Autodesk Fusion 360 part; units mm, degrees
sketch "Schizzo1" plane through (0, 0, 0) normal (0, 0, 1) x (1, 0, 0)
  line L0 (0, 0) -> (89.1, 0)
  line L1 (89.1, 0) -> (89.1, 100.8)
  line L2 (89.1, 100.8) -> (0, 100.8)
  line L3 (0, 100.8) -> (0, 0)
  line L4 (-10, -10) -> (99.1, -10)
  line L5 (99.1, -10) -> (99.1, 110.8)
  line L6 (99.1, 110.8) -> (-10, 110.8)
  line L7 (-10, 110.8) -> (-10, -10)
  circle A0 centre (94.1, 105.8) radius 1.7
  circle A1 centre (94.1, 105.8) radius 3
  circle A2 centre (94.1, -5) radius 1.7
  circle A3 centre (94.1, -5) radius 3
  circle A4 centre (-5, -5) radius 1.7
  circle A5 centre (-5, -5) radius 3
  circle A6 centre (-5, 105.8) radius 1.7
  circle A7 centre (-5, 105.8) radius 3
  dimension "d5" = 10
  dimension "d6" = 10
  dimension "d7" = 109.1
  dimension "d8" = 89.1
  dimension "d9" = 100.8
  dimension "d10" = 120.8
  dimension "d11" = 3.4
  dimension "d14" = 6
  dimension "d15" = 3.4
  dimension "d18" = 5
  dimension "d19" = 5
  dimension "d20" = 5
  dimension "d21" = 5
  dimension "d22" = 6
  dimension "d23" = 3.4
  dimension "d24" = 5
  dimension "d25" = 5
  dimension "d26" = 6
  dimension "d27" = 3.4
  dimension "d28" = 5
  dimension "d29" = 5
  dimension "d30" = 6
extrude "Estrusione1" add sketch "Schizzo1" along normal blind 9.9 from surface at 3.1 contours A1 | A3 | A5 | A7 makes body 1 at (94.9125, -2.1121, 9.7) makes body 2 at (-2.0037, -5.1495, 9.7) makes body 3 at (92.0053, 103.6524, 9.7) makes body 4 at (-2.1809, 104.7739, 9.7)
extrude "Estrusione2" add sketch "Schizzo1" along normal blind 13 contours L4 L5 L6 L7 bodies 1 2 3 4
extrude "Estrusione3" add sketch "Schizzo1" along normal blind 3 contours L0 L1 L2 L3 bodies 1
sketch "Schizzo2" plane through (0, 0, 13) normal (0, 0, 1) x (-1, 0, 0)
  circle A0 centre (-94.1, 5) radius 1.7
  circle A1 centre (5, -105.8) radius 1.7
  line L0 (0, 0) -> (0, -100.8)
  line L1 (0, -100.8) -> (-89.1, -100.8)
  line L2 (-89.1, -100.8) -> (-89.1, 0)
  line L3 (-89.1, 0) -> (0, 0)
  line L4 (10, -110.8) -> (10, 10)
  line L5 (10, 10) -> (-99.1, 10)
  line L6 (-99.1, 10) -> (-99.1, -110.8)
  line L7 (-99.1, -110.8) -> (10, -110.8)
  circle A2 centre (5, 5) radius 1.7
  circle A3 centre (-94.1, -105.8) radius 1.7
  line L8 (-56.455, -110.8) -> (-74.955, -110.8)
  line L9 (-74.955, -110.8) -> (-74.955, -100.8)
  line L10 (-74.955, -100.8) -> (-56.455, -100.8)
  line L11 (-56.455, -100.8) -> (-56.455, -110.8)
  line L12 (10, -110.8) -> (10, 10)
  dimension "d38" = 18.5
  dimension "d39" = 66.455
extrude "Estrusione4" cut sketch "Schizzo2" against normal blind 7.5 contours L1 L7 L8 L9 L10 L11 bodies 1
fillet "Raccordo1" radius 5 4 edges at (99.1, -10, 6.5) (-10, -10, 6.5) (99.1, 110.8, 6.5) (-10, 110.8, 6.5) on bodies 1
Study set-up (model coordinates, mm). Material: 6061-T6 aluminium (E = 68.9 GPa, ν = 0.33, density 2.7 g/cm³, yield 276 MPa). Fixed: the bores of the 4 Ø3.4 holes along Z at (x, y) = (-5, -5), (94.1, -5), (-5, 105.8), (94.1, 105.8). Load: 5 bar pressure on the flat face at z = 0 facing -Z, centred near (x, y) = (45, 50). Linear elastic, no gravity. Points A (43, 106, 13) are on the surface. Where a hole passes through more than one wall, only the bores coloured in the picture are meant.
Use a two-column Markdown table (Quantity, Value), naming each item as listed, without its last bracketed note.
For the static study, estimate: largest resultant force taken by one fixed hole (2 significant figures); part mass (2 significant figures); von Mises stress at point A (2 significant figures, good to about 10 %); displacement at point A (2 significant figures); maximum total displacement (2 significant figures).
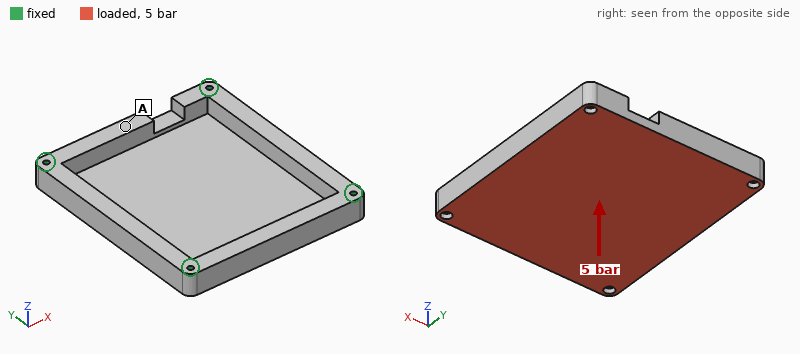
| Quantity | Value |
|---|---|
| largest resultant force taken by one fixed hole | 2.8 kN |
| part mass | 210 g |
| von Mises stress at point A | 21 MPa |
| displacement at point A | 0.083 mm |
| maximum total displacement | 0.50 mm |
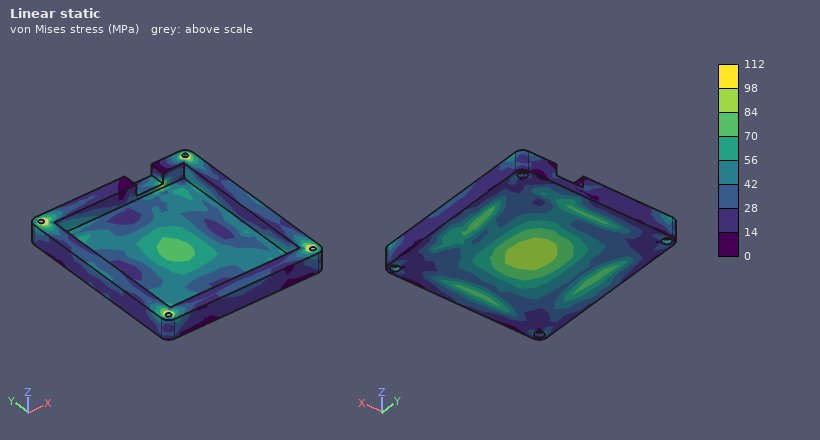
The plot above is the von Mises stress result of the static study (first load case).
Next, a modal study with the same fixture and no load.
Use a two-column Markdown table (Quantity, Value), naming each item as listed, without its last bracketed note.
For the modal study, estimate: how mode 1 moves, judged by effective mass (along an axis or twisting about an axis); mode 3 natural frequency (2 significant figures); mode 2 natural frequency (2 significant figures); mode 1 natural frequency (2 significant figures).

| Quantity | Value |
|---|---|
| how mode 1 moves, judged by effective mass | along Z |
| mode 3 natural frequency | 4000 Hz |
| mode 2 natural frequency | 3900 Hz |
| mode 1 natural frequency | 2300 Hz |
